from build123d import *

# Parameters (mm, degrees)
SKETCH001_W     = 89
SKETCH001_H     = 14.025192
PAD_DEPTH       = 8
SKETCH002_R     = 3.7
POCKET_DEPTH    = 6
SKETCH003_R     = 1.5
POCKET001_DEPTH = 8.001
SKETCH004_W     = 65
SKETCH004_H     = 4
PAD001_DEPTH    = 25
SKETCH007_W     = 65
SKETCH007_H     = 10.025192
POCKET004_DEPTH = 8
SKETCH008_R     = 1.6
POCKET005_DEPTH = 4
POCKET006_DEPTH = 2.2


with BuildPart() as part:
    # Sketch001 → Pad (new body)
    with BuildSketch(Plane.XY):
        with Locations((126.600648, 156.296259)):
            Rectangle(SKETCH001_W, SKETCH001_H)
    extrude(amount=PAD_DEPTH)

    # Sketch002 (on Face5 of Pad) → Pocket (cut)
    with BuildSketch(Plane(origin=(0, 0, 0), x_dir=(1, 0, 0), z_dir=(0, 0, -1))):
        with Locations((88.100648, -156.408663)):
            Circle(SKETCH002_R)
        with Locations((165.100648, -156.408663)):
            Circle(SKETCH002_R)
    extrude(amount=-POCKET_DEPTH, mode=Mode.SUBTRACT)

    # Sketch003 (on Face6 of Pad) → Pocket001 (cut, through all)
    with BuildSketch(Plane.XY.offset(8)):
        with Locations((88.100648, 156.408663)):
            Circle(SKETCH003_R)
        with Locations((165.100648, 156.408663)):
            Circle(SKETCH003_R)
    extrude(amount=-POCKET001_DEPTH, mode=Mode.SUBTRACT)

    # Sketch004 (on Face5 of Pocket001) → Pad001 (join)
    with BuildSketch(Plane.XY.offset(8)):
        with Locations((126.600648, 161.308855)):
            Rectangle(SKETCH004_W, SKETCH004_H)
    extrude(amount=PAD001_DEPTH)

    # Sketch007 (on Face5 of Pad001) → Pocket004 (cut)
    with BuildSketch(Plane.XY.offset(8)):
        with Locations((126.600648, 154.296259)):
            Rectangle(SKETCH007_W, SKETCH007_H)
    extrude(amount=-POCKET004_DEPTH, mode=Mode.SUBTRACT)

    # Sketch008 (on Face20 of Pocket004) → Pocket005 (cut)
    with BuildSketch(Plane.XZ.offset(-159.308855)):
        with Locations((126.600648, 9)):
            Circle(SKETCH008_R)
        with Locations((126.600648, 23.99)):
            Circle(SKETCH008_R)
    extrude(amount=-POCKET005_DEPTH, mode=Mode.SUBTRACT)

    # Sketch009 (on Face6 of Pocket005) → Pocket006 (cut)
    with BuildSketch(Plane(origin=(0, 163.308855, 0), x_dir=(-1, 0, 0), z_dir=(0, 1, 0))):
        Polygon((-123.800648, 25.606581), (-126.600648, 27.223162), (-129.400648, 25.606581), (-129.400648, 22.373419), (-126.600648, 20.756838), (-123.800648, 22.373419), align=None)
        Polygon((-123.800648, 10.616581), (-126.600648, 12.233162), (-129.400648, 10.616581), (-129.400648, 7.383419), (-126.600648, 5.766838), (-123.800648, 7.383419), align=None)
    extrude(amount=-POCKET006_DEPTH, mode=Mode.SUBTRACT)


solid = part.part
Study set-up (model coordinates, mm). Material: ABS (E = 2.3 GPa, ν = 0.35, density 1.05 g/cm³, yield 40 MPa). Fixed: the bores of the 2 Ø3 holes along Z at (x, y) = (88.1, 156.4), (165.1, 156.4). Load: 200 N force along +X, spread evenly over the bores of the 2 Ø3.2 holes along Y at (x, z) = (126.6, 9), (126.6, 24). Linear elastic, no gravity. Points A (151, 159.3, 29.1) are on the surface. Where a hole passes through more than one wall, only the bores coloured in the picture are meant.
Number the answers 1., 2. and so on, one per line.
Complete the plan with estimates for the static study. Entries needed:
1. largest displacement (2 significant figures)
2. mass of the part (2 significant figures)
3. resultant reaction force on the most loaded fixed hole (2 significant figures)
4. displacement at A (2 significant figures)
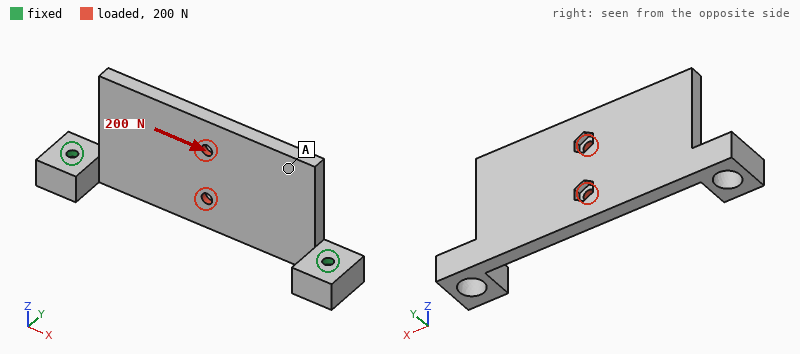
1. 0.22 mm
2. 11 g
3. 100 N
4. 0.19 mm
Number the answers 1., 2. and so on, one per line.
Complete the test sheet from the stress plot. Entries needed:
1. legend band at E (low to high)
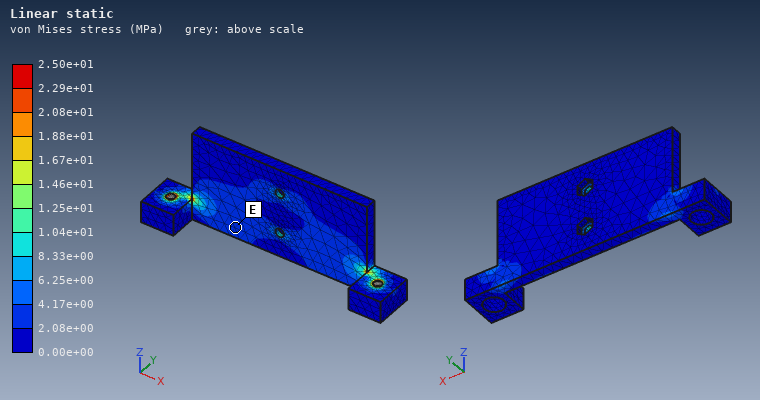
1. 2.08e+00 to 4.17e+00 MPa
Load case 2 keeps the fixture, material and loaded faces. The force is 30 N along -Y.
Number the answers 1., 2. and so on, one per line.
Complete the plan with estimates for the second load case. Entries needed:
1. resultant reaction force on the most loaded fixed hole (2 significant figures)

1. 29 N
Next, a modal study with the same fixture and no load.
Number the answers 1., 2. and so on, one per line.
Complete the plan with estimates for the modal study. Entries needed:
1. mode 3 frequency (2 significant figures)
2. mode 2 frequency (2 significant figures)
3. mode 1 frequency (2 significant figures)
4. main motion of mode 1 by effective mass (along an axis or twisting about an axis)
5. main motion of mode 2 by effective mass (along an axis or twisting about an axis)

1. 1200 Hz
2. 1100 Hz
3. 440 Hz
4. along Y
5. along Y
